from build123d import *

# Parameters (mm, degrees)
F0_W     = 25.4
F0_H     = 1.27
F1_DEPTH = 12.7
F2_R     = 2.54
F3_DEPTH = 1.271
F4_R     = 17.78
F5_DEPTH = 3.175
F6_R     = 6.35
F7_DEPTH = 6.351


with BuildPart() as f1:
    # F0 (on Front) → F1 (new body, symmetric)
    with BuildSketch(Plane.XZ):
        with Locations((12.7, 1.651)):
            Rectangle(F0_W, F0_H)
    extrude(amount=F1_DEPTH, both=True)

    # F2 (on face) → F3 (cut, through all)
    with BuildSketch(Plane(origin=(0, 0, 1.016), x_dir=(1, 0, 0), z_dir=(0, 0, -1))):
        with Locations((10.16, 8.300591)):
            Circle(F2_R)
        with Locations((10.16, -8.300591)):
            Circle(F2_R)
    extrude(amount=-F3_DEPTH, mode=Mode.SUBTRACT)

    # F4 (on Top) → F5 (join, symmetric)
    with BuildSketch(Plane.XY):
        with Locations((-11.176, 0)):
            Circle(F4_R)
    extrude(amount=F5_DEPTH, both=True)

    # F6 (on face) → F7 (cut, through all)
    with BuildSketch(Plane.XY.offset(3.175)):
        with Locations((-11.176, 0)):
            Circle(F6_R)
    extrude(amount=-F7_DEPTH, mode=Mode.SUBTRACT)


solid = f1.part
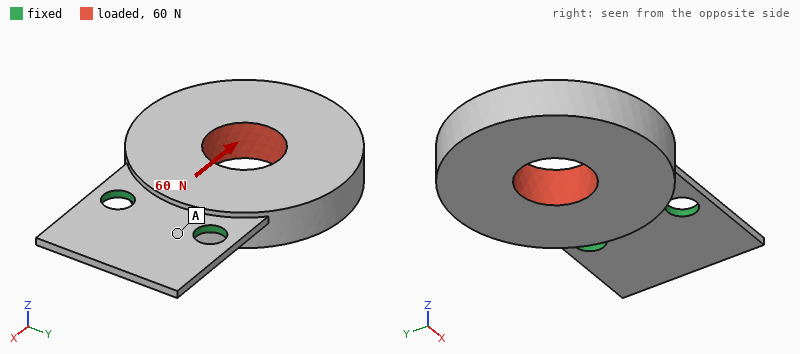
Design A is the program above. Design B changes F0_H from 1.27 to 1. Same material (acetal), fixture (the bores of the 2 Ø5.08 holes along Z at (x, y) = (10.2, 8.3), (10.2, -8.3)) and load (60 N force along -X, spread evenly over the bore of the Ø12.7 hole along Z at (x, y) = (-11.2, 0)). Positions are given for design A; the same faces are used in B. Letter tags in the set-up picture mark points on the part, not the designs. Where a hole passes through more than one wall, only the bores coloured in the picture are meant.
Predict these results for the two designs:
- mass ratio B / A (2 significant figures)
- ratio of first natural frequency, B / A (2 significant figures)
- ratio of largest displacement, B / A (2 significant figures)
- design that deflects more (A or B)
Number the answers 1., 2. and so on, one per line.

1. 0.98
2. 0.73
3. 1.9
4. B
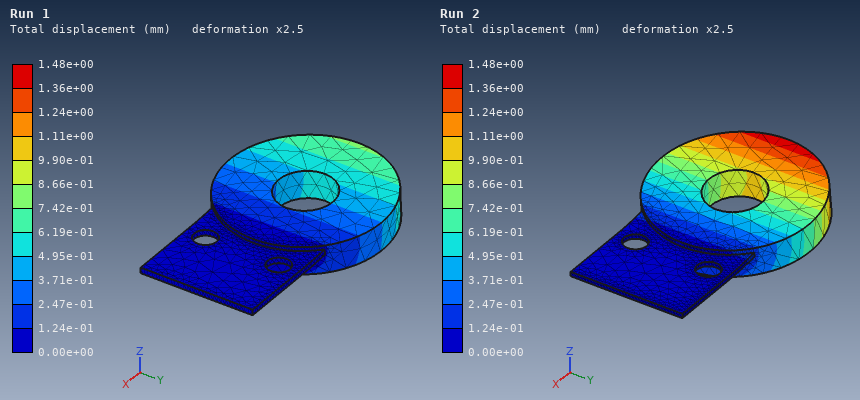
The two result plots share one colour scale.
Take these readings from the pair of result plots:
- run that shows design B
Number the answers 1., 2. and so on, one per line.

1. Run 2
